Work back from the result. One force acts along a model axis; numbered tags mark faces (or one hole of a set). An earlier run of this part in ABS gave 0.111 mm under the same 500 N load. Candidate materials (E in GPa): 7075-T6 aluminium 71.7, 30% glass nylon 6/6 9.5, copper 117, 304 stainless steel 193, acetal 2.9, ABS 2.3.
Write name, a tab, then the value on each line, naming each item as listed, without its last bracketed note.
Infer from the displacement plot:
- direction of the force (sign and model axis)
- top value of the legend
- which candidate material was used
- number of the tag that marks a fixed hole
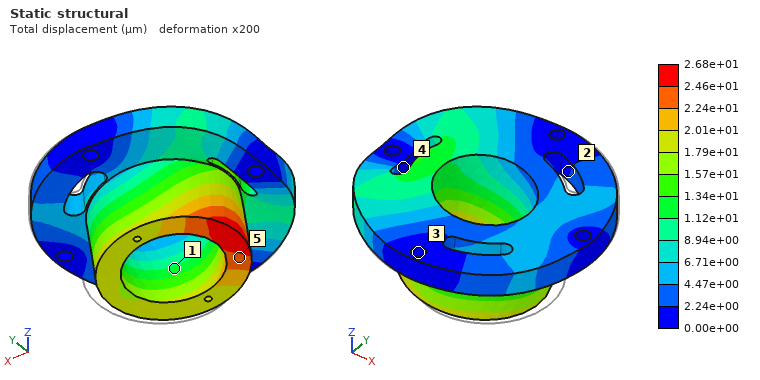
direction of the force	-X
top value of the legend	2.68e+01 µm
which candidate material was used	30% glass nylon 6/6
number of the tag that marks a fixed hole	3
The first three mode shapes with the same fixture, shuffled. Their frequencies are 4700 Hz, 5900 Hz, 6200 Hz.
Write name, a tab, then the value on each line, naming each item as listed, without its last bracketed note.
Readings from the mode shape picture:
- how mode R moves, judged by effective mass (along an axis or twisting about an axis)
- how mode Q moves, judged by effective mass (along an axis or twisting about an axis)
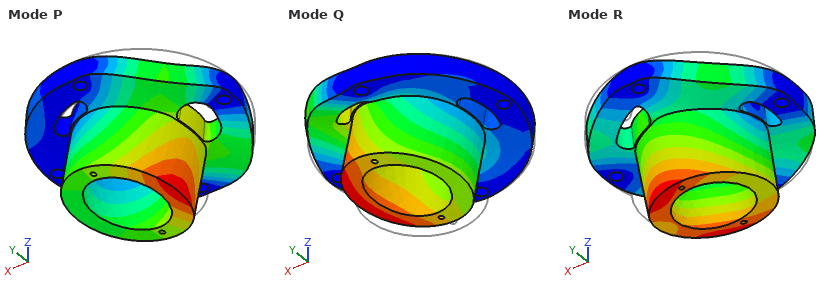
how mode R moves, judged by effective mass	along Y
how mode Q moves, judged by effective mass	along Z
